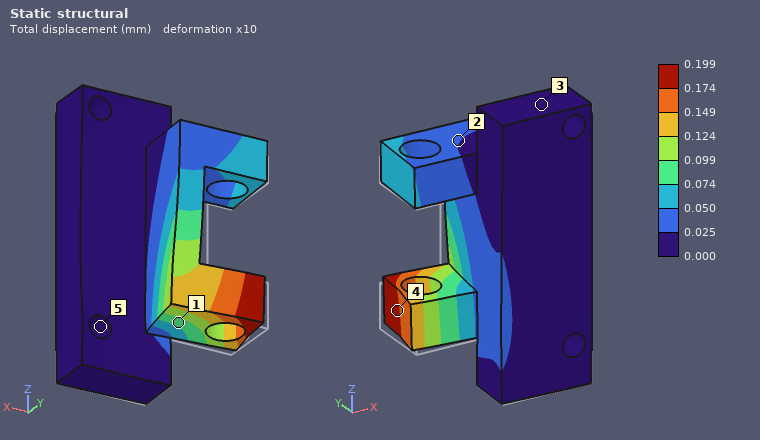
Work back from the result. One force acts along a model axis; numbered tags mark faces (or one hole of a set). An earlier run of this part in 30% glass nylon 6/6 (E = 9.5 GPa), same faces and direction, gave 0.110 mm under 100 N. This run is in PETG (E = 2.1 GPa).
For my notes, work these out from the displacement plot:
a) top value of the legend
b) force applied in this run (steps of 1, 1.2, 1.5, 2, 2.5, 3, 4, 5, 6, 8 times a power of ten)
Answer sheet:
0.199 mm
40 N
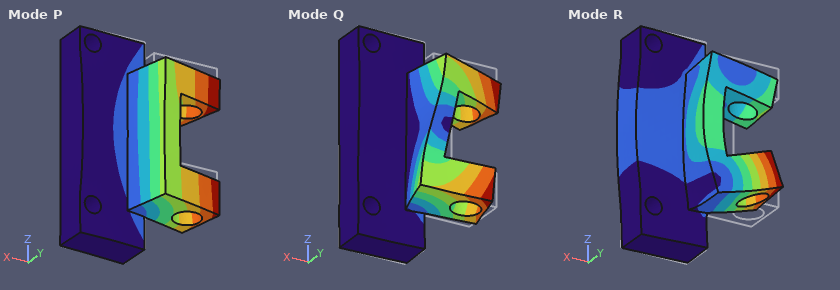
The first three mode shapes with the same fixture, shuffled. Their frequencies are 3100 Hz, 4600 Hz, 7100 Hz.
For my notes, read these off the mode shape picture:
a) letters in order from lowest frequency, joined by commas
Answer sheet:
P, Q, R
